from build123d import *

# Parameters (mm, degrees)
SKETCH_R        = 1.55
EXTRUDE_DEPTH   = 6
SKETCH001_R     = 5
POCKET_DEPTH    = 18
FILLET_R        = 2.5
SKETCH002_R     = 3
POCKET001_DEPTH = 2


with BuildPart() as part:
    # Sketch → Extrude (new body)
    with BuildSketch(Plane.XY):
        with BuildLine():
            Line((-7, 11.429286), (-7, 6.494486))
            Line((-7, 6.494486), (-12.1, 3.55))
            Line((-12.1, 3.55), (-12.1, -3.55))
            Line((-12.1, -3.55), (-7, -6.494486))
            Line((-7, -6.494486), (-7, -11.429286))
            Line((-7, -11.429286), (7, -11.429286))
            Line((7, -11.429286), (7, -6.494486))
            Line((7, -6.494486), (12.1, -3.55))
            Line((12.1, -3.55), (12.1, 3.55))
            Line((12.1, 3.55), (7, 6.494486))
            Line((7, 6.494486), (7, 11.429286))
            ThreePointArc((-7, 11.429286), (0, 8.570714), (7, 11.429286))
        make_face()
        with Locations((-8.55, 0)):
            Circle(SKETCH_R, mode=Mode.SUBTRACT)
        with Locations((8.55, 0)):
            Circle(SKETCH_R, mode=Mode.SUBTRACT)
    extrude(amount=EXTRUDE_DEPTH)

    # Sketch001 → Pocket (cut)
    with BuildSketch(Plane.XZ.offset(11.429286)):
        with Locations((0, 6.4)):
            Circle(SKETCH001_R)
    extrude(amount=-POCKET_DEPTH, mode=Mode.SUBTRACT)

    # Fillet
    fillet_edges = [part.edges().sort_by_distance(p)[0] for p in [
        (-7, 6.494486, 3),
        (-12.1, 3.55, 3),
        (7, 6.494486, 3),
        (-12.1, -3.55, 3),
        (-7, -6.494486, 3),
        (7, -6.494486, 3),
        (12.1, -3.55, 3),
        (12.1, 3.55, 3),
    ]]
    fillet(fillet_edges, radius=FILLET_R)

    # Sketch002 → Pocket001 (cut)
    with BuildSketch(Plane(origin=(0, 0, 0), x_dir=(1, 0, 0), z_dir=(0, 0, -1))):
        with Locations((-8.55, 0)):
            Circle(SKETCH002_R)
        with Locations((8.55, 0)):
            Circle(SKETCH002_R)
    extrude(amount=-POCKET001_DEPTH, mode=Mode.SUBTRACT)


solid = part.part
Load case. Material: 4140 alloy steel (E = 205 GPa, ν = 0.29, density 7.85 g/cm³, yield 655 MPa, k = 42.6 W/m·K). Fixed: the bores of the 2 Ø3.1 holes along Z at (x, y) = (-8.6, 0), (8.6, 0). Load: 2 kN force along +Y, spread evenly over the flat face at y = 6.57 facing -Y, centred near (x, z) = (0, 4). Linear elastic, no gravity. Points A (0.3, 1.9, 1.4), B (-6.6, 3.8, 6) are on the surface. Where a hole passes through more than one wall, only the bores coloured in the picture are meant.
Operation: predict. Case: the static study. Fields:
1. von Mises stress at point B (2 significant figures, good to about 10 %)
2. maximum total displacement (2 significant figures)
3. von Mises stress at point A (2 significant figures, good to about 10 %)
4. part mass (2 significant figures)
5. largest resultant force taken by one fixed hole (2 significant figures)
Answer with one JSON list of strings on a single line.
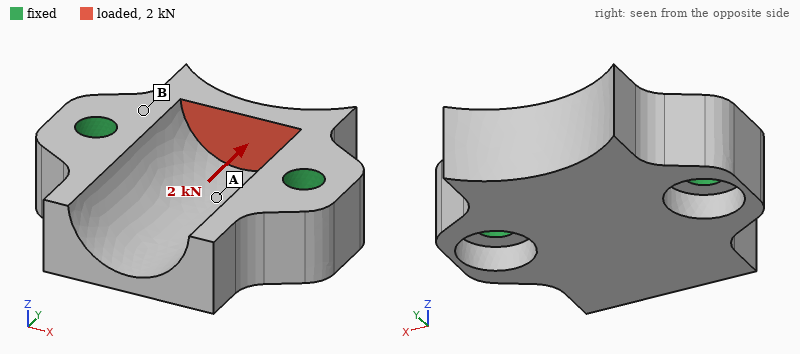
["100 MPa", "17 µm", "40 MPa", "12 g", "1.1 kN"]
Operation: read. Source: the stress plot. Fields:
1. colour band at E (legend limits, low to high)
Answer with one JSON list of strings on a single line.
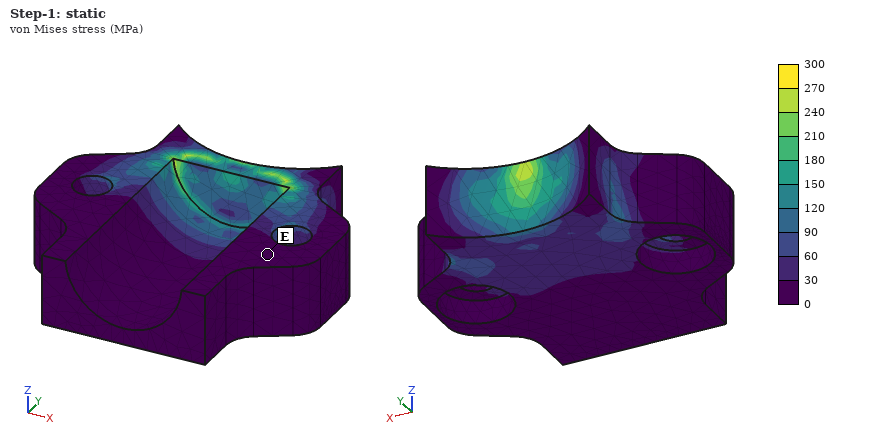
["0 to 30 MPa"]
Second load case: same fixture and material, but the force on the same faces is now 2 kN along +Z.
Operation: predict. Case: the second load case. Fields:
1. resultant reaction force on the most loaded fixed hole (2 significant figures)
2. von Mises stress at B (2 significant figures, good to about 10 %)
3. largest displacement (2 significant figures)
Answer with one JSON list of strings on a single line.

["1.1 kN", "140 MPa", "21 µm"]
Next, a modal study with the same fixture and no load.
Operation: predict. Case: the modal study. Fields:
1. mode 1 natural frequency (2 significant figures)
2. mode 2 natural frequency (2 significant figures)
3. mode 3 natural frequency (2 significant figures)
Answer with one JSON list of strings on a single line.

["26 kHz", "36 kHz", "37 kHz"]
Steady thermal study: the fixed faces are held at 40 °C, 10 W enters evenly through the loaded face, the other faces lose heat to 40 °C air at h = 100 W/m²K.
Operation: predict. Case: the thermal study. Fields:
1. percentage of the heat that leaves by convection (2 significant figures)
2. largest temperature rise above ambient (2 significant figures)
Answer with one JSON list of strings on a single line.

["13 %", "51 K"]
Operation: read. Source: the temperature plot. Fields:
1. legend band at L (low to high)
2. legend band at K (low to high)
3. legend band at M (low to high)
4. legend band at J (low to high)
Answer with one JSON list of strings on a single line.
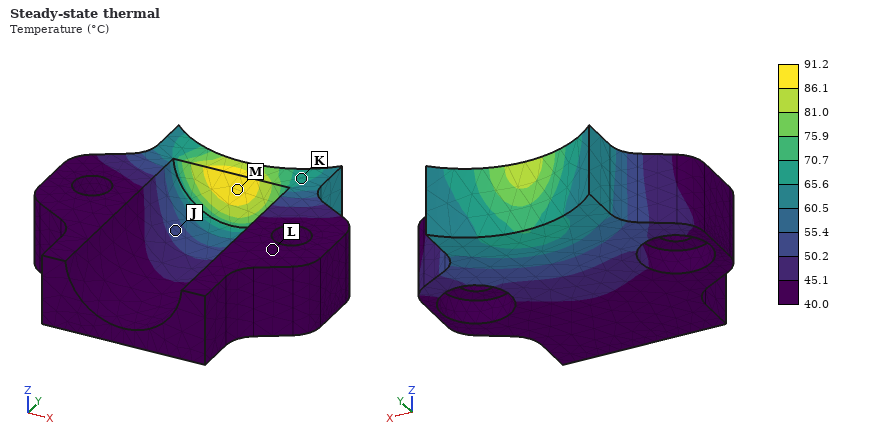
["40.0 to 45.1 °C", "65.6 to 70.7 °C", "86.1 to 91.2 °C", "50.2 to 55.4 °C"]
